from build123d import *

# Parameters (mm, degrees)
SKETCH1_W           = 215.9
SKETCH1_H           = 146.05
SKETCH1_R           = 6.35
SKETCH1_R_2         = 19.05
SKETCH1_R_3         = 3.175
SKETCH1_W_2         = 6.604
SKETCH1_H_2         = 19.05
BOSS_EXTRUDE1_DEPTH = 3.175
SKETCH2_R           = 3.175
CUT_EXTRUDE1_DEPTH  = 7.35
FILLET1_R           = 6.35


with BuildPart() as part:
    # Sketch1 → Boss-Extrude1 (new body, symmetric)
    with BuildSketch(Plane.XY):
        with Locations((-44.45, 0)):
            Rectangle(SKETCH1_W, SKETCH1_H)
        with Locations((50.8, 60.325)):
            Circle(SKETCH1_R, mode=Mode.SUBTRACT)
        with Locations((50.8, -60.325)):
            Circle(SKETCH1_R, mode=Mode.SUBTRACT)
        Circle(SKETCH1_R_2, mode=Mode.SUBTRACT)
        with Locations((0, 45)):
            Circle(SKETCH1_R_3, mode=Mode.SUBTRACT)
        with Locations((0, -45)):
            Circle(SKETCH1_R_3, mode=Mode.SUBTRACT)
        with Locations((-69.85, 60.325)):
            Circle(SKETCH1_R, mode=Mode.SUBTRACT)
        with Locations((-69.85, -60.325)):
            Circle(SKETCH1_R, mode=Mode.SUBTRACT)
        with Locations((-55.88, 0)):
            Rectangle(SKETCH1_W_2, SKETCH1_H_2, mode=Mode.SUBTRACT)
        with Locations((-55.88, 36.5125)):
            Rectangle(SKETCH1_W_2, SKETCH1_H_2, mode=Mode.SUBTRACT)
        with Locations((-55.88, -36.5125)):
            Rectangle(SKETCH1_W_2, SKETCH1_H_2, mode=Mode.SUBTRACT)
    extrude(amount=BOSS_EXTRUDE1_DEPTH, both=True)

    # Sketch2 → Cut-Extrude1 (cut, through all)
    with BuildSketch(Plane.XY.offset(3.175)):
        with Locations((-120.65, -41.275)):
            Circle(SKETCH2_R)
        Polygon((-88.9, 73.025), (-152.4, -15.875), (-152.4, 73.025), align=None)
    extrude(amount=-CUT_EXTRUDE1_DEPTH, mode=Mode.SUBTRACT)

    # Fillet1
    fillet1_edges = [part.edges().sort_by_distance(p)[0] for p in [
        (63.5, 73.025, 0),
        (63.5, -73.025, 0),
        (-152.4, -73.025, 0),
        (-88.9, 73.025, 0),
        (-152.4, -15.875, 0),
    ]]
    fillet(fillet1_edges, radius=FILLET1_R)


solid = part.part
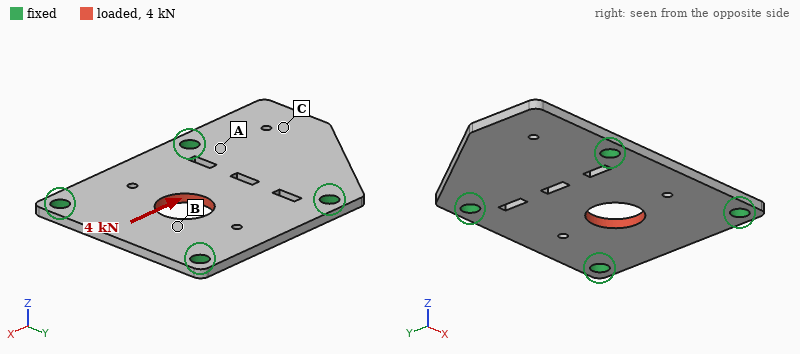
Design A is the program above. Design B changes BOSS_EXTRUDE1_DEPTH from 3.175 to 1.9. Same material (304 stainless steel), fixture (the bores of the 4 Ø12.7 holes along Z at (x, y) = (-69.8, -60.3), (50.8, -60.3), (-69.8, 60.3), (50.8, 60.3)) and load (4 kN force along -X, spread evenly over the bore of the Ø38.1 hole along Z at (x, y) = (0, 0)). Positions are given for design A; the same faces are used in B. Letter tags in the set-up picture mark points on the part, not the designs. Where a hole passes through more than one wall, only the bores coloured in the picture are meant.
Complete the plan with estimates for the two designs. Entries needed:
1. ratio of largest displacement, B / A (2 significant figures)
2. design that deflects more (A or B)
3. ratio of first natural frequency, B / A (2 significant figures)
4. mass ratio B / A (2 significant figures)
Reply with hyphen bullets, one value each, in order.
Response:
- 1.7
- B
- 0.61
- 0.60
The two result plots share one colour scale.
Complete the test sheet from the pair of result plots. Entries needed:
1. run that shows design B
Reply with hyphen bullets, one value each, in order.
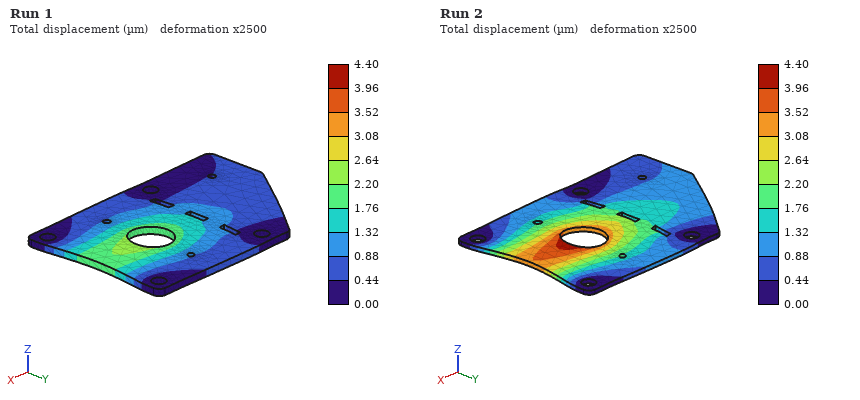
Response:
- Run 2
